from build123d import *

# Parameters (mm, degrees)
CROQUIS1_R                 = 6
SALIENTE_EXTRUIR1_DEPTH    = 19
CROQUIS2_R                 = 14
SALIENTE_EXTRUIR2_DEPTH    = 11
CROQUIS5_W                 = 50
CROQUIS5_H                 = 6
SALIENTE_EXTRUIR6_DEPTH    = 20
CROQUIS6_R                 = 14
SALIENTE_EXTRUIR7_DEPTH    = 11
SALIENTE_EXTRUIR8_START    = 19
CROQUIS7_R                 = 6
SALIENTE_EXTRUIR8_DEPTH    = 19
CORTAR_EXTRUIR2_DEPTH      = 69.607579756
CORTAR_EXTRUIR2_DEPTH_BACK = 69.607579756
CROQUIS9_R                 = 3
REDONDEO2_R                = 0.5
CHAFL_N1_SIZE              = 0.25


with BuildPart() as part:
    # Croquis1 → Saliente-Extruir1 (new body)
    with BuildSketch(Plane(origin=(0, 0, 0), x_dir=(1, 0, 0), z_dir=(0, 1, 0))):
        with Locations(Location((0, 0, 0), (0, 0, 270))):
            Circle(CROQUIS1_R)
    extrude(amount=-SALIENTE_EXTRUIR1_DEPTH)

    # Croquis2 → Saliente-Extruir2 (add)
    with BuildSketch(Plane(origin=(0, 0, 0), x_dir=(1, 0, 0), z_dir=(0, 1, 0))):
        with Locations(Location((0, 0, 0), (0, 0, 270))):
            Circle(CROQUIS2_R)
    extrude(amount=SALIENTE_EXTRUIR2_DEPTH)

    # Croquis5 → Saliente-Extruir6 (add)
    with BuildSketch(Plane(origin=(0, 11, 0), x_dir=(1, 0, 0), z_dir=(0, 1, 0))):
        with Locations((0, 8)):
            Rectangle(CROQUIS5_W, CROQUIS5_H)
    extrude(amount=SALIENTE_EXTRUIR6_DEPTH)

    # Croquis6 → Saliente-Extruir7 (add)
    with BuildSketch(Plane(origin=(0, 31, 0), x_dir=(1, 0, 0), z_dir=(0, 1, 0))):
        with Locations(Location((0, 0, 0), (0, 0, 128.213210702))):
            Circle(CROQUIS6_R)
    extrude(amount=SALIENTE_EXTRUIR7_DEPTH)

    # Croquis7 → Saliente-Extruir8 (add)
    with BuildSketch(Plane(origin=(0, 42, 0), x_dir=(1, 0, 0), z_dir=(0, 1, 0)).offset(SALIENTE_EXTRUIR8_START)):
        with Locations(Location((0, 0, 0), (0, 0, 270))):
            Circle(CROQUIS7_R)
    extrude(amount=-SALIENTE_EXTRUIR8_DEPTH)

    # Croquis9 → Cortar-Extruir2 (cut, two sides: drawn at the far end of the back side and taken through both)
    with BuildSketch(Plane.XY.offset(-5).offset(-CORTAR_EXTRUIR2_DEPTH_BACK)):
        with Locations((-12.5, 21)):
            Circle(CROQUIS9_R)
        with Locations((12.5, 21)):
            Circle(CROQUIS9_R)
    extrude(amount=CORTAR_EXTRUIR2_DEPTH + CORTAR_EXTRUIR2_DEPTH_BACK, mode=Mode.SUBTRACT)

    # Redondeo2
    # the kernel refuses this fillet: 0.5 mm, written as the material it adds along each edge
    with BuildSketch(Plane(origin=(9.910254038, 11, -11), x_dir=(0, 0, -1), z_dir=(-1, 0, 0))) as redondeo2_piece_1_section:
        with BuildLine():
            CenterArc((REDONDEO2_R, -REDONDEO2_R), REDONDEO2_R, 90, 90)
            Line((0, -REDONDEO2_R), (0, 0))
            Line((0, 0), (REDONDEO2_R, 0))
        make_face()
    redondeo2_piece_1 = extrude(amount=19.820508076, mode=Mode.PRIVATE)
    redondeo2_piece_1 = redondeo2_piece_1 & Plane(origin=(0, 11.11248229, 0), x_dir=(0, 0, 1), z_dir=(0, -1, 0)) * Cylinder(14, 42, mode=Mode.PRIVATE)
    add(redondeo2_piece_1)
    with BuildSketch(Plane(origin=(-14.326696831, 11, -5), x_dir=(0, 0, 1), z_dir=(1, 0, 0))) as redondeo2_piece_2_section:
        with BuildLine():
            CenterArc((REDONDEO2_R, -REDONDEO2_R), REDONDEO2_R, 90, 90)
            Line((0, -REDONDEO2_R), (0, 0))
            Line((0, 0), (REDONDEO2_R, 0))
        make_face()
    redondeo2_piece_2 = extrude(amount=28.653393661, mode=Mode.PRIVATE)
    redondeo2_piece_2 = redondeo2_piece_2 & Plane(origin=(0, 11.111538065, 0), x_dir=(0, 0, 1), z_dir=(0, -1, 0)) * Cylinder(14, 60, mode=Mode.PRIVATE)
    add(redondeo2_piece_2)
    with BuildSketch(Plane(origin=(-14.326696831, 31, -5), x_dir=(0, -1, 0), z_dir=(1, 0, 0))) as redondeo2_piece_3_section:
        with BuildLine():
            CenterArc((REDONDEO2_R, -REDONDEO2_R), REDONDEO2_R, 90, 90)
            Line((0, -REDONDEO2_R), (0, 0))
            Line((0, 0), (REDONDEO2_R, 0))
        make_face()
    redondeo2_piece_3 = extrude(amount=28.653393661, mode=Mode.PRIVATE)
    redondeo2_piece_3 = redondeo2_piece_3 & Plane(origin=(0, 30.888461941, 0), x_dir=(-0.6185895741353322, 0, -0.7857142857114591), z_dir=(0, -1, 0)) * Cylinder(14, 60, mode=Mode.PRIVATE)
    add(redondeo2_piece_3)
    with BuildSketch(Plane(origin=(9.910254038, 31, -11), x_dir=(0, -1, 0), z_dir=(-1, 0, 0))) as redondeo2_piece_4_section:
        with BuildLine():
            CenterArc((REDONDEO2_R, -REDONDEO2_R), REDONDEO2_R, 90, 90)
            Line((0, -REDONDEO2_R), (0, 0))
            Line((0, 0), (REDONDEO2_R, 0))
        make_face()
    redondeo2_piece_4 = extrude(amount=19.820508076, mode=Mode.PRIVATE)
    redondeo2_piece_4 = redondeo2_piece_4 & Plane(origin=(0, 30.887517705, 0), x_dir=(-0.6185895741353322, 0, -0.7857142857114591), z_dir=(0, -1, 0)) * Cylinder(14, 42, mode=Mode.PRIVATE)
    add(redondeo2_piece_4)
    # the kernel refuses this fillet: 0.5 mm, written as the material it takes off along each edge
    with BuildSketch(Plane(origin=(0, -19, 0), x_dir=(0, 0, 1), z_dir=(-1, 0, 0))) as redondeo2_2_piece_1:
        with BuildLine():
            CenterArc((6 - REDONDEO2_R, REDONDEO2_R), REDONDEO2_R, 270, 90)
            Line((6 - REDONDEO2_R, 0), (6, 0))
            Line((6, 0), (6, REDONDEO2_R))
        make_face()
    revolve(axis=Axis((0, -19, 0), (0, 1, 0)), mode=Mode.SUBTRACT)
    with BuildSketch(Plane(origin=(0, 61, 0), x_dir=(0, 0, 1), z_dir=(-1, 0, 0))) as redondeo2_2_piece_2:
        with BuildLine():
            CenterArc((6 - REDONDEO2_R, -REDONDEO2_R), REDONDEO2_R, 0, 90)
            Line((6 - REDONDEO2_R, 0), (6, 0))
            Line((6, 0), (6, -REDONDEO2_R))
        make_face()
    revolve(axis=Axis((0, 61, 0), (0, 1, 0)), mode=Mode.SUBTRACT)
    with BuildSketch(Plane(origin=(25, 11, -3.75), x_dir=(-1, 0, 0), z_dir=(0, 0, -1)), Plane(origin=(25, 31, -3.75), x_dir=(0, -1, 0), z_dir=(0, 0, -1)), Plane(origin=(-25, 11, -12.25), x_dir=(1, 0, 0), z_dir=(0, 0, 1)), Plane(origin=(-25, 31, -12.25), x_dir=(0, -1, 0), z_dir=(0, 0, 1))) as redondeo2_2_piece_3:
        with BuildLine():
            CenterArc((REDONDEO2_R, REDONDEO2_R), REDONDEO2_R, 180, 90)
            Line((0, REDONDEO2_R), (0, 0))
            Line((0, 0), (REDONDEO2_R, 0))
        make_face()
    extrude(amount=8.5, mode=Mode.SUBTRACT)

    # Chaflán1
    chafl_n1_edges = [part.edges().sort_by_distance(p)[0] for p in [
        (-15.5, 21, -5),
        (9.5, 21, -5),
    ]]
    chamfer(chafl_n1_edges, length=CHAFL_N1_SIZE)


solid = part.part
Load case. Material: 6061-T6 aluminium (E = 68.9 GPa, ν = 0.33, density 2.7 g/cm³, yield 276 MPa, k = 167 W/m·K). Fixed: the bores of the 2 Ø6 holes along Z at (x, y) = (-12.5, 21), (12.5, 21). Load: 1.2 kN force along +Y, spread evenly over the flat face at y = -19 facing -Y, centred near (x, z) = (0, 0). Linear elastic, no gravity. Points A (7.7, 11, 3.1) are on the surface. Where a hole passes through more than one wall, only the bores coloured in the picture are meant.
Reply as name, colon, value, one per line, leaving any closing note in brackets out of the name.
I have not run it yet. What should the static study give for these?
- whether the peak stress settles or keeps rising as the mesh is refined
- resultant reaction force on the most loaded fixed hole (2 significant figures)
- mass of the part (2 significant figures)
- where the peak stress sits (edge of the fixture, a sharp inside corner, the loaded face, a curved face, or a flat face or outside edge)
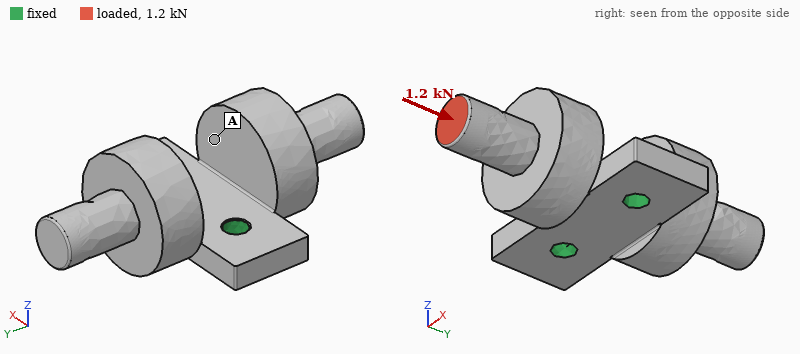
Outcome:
whether the peak stress settles or keeps rising as the mesh is refined: keeps rising
resultant reaction force on the most loaded fixed hole: 620 N
mass of the part: 63 g
where the peak stress sits: a sharp inside corner
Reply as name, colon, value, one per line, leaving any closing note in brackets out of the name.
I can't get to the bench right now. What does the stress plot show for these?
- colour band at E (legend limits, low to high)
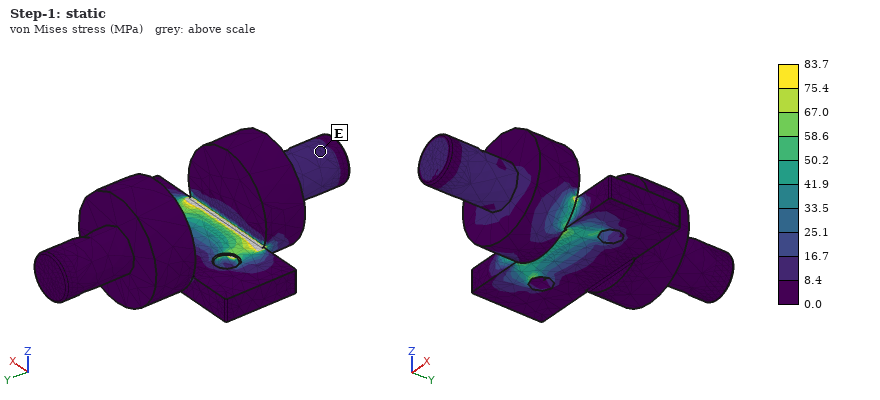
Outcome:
colour band at E: 8.4 to 16.7 MPa
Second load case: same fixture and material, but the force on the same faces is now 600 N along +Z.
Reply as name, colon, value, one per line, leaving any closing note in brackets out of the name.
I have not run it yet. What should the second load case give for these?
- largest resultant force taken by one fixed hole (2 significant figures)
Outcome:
largest resultant force taken by one fixed hole: 300 N
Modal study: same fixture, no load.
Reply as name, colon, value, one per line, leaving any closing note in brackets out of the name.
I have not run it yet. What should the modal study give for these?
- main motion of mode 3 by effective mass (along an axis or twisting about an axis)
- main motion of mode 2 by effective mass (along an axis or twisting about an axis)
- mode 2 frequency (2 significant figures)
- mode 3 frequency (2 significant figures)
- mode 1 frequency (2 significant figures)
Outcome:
main motion of mode 3 by effective mass: twisting about Z
main motion of mode 2 by effective mass: along Z
mode 2 frequency: 3200 Hz
mode 3 frequency: 9300 Hz
mode 1 frequency: 3000 Hz
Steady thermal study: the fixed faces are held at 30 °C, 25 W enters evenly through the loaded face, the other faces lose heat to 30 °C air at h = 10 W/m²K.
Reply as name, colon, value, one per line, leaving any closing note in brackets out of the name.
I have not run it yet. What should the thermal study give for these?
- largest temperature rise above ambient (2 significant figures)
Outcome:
largest temperature rise above ambient: 43 K
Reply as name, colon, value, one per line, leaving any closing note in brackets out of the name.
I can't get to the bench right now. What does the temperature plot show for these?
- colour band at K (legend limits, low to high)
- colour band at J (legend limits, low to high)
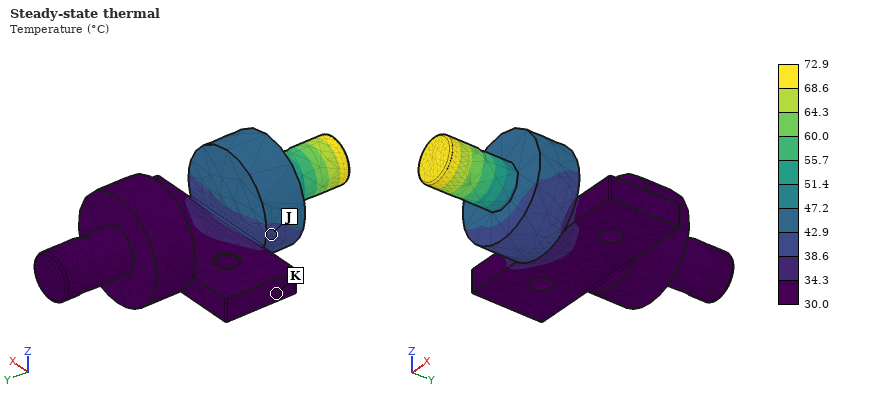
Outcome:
colour band at K: 30.0 to 34.3 °C
colour band at J: 38.6 to 42.9 °C
